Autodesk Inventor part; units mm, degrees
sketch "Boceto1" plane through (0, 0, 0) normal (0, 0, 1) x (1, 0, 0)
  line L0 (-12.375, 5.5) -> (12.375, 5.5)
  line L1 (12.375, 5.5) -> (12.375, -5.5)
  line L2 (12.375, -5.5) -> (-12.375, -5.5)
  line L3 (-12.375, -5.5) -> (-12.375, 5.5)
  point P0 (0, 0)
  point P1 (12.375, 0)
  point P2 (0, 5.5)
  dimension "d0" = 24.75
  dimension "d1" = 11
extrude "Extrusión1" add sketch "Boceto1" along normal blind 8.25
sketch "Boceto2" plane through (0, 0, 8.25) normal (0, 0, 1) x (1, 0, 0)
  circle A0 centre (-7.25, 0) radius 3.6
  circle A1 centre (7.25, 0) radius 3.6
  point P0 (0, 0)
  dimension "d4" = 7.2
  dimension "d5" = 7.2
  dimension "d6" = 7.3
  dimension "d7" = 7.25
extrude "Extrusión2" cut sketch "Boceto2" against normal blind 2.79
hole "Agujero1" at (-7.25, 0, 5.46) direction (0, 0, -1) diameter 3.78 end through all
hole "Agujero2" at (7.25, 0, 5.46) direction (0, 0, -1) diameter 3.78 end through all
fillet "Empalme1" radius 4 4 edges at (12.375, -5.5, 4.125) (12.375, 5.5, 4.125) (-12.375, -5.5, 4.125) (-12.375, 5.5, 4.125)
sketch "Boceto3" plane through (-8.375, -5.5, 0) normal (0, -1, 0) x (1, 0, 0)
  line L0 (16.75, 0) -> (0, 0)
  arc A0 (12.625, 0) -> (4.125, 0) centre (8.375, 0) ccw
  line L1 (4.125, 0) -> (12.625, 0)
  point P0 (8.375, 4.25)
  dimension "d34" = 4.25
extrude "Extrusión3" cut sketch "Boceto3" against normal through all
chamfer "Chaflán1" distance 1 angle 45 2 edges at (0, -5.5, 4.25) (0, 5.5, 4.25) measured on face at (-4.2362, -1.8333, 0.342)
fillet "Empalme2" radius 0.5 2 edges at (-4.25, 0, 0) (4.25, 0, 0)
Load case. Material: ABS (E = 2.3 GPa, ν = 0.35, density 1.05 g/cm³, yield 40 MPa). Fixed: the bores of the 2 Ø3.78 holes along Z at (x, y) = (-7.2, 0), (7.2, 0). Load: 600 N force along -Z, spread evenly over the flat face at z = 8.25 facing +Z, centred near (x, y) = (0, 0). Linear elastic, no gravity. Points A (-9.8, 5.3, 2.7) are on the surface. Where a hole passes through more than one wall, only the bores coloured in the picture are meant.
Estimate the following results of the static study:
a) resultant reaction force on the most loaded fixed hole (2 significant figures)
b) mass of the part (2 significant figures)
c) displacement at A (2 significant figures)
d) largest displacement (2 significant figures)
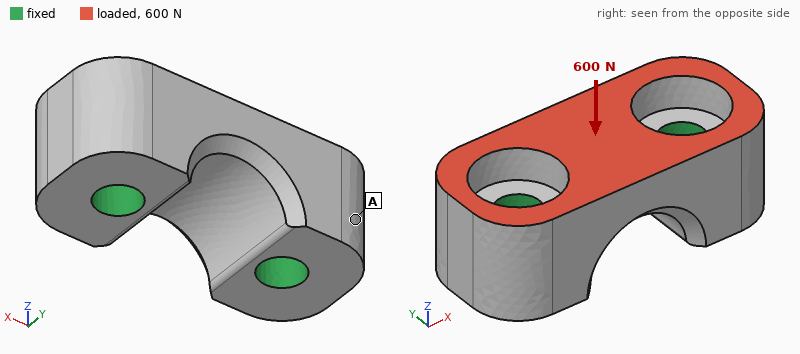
310 N
1.5 g
11 µm
35 µm
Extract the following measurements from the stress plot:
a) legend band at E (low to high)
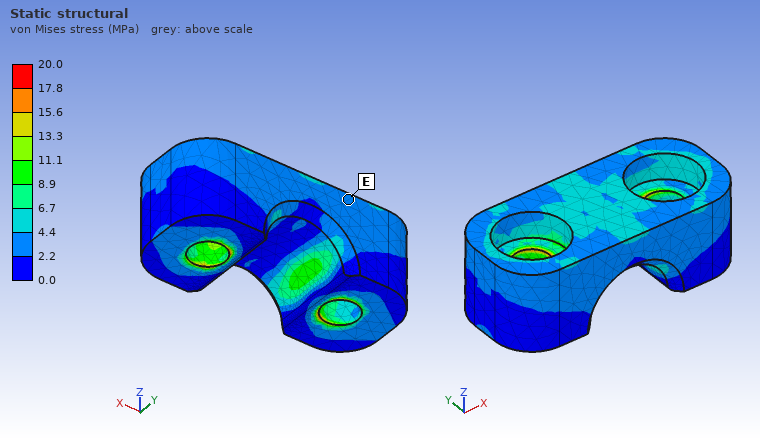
2.2 to 4.4 MPa
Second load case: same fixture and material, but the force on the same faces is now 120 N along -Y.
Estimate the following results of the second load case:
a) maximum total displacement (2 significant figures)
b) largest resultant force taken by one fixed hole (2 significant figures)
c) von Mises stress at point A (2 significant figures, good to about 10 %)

27 µm
60 N
0.96 MPa
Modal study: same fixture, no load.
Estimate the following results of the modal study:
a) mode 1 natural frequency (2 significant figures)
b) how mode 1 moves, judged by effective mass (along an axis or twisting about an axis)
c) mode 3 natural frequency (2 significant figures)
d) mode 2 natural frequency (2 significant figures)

18 kHz
along Y
25 kHz
25 kHz
